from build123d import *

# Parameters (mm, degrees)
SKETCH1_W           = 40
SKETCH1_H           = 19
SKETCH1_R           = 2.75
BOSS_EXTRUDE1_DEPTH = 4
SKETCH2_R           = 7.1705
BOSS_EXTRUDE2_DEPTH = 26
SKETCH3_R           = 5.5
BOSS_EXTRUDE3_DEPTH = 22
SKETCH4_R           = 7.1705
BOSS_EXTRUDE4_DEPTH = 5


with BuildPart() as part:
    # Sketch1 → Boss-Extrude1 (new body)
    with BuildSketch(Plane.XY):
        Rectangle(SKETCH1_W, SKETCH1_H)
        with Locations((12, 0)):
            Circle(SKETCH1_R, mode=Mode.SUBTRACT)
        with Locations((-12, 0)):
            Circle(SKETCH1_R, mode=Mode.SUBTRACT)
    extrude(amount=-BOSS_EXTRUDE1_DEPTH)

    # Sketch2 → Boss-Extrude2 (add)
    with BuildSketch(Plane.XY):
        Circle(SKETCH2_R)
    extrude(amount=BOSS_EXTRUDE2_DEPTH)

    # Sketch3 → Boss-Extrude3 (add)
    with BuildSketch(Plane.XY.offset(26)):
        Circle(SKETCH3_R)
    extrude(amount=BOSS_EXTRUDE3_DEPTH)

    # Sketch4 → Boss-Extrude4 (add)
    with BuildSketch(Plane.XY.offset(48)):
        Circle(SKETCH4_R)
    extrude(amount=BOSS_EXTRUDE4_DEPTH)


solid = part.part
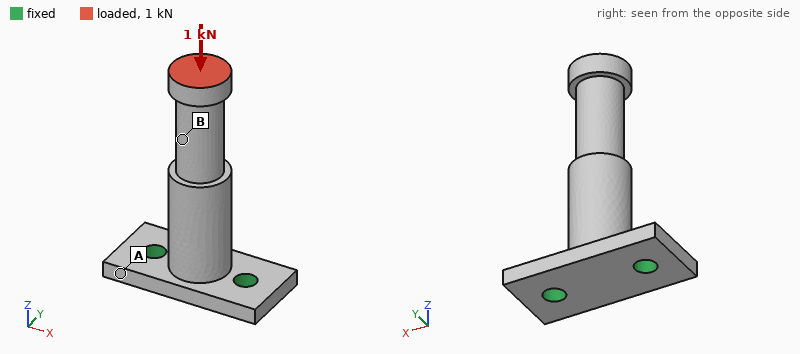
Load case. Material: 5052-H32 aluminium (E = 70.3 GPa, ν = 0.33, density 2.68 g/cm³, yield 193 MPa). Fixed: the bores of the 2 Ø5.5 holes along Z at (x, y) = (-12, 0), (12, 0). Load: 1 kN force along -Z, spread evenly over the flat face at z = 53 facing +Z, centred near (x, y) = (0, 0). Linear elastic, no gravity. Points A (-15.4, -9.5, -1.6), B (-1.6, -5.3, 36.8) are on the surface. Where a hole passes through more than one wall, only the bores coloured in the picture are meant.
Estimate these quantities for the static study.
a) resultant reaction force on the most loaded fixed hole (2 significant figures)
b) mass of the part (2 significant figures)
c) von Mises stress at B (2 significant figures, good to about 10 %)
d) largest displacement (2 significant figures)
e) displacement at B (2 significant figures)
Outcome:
530 N
27 g
10 MPa
10 µm
7.7 µm
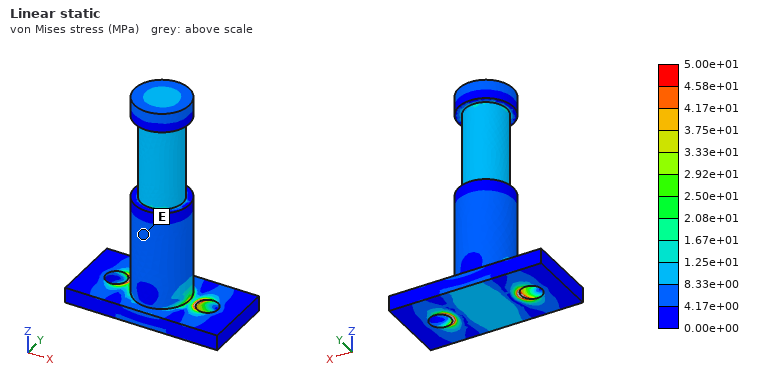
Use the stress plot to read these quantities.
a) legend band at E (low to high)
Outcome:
4.17e+00 to 8.33e+00 MPa
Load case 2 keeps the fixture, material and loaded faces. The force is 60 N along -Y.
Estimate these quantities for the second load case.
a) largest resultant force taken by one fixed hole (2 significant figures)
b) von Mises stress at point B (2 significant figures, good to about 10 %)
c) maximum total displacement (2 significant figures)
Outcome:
30 N
7.1 MPa
72 µm
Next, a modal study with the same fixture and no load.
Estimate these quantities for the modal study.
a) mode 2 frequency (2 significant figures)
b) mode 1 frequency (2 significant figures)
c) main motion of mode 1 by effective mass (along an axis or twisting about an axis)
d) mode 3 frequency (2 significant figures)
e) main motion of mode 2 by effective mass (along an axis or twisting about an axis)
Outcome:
3200 Hz
2100 Hz
along Y
12 kHz
along X
